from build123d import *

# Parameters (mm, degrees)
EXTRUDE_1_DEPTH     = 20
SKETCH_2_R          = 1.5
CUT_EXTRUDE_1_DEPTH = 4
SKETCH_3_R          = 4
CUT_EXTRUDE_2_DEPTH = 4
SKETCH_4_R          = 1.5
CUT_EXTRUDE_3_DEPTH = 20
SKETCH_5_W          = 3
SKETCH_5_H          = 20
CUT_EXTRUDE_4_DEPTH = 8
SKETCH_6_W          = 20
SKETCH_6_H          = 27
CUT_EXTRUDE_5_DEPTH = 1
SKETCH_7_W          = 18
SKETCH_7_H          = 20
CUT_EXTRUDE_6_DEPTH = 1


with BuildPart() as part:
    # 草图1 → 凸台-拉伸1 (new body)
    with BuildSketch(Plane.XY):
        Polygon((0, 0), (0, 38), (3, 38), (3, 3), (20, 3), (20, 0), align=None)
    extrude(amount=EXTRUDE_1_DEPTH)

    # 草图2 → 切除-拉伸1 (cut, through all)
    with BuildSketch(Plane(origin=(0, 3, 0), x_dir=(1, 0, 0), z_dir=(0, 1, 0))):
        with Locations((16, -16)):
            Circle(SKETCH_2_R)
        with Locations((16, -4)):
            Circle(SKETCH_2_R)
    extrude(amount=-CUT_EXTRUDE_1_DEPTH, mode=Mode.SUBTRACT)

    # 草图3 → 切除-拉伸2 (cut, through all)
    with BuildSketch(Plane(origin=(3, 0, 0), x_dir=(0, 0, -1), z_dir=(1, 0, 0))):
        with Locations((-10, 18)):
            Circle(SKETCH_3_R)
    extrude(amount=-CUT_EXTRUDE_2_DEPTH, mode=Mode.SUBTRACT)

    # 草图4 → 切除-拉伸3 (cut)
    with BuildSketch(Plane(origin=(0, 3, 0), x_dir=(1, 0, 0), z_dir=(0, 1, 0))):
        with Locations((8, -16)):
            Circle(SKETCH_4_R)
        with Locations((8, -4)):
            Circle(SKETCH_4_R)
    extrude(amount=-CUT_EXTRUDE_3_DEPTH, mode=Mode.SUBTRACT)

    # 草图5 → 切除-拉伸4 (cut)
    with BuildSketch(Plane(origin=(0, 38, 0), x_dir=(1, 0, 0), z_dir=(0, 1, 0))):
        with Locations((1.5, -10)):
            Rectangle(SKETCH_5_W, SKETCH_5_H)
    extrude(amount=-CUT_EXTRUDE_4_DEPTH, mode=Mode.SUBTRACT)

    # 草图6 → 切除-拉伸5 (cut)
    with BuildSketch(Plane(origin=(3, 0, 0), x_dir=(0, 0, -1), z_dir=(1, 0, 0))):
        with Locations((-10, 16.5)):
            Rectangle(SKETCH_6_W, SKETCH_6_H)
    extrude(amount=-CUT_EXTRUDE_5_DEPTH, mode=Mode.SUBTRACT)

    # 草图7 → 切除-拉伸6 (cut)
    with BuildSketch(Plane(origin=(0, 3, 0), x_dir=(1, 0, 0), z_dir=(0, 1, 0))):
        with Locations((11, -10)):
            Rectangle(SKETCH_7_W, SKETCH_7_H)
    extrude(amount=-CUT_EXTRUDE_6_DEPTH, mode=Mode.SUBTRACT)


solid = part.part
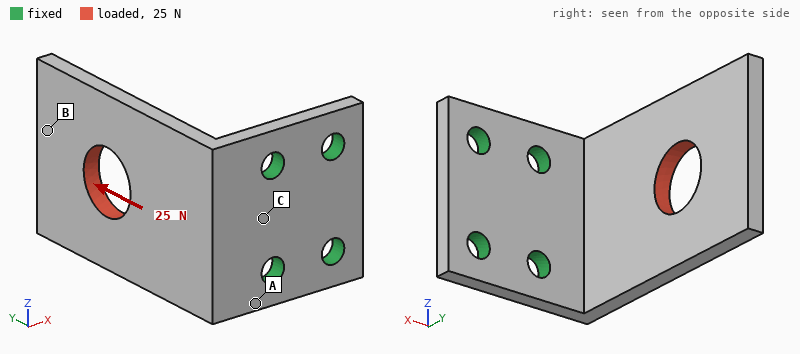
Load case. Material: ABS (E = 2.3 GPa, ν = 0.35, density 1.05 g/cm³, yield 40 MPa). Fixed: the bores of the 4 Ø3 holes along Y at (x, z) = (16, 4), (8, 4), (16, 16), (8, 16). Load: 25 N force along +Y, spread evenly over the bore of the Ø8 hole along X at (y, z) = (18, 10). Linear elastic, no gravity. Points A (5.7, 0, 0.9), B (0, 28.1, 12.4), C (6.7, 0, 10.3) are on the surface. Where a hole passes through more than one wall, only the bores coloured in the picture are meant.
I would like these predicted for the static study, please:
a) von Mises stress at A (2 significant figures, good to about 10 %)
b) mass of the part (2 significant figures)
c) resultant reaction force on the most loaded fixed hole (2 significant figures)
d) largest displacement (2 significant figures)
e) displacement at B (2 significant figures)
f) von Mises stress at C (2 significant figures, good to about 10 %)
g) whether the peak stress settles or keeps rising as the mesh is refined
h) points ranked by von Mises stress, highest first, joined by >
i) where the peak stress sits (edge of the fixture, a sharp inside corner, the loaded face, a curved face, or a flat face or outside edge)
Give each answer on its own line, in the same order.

7.0 MPa
1.9 g
14 N
0.46 mm
0.43 mm
4.5 MPa
keeps rising
A > C > B
edge of the fixture
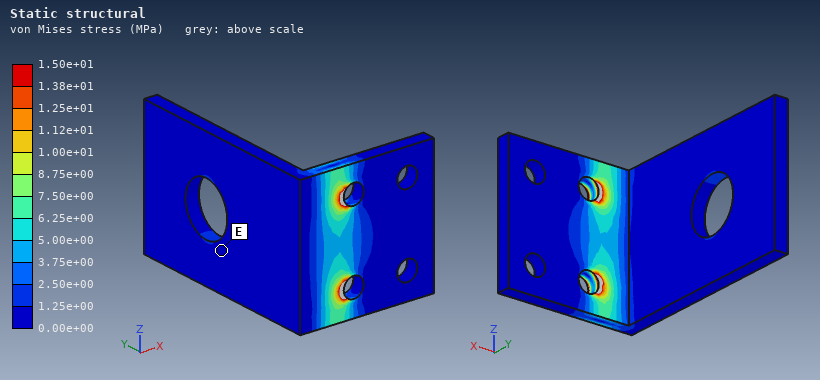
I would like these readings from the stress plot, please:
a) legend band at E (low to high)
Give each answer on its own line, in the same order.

0.00e+00 to 1.25e+00 MPa
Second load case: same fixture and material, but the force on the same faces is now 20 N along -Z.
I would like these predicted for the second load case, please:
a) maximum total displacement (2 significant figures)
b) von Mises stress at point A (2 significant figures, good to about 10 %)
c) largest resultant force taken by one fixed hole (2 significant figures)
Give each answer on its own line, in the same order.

0.43 mm
9.7 MPa
29 N
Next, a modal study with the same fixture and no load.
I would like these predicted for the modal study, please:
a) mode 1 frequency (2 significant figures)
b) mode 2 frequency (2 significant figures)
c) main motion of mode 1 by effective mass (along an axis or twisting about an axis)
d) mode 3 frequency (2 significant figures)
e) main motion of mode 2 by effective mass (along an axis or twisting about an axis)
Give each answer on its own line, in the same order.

450 Hz
1300 Hz
along X
1700 Hz
along Z
